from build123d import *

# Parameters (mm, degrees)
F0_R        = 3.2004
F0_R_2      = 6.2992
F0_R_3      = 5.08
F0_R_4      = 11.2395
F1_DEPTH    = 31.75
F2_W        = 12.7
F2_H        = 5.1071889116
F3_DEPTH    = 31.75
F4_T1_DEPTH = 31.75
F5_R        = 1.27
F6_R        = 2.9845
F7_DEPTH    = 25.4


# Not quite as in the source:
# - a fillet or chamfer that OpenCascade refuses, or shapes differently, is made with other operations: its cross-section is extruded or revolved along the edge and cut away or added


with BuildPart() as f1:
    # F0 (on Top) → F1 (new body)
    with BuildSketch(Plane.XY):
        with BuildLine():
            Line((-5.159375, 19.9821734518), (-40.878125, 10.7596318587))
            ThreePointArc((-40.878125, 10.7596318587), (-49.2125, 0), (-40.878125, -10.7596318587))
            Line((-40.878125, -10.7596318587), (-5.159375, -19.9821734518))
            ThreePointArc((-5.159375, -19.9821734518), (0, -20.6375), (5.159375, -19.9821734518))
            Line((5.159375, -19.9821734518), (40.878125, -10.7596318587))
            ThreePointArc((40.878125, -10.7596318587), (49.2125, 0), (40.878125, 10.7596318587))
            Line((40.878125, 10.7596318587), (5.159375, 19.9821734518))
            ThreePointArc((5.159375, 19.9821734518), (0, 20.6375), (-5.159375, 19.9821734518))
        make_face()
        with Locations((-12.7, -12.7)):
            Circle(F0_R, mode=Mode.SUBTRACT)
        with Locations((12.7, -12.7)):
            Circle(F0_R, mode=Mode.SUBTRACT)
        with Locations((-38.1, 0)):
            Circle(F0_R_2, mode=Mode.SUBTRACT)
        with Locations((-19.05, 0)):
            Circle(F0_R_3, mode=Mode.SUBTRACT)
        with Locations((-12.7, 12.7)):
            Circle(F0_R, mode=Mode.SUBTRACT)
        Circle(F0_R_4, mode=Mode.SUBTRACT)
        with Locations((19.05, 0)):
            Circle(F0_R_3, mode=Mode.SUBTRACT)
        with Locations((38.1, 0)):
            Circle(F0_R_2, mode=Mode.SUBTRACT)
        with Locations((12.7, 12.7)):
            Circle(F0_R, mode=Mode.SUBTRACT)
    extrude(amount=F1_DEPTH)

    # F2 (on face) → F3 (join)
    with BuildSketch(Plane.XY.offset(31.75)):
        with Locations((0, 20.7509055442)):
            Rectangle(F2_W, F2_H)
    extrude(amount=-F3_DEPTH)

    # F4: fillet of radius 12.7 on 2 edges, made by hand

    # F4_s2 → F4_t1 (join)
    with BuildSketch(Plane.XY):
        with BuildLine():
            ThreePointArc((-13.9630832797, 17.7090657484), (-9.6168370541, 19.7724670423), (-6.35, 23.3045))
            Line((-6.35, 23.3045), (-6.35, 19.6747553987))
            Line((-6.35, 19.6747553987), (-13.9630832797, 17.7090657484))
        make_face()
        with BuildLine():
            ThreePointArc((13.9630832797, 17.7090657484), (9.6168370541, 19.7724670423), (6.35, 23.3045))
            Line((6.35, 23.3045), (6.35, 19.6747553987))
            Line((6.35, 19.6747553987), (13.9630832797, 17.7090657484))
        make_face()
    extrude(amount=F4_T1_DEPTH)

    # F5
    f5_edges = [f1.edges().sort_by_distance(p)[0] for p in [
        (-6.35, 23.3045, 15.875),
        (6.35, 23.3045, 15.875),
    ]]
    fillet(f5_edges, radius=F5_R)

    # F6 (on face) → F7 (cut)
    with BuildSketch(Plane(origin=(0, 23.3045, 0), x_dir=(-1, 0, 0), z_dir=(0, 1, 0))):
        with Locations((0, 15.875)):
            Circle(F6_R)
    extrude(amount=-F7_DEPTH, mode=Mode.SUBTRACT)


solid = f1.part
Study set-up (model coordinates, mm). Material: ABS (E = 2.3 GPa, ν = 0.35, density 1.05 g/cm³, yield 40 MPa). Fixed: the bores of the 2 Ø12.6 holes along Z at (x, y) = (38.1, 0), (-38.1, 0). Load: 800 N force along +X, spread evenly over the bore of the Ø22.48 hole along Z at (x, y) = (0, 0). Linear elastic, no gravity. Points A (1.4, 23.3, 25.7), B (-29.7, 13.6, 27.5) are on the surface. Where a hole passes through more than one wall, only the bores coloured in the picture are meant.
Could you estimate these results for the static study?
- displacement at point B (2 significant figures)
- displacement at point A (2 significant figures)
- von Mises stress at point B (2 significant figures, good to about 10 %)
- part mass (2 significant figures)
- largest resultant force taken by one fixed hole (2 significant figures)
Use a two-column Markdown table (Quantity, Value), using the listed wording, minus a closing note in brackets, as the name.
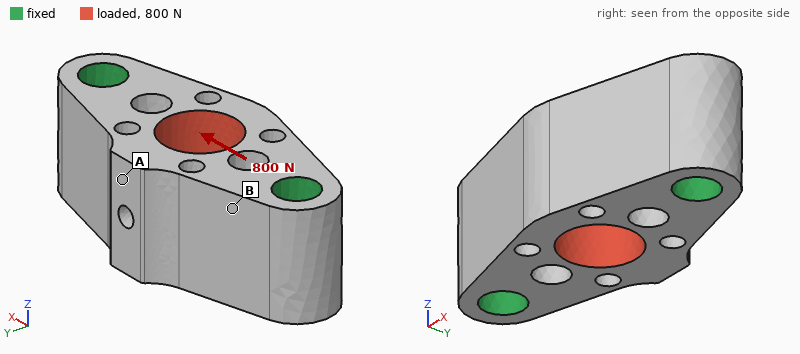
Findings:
| Quantity | Value |
|---|---|
| displacement at point B | 3.9 µm |
| displacement at point A | 5.6 µm |
| von Mises stress at point B | 0.43 MPa |
| part mass | 66 g |
| largest resultant force taken by one fixed hole | 400 N |
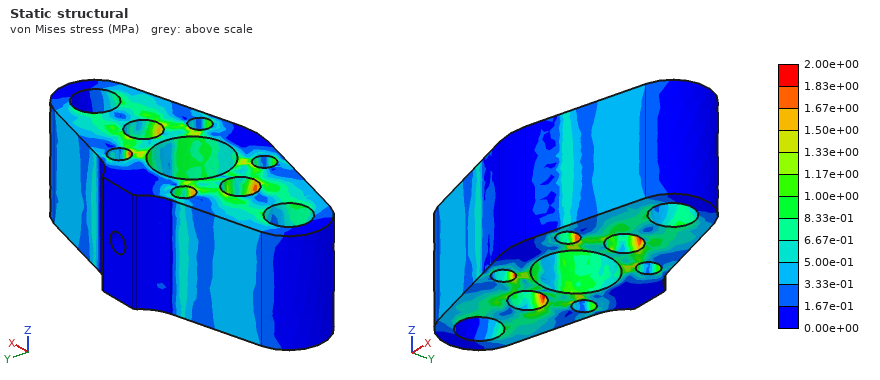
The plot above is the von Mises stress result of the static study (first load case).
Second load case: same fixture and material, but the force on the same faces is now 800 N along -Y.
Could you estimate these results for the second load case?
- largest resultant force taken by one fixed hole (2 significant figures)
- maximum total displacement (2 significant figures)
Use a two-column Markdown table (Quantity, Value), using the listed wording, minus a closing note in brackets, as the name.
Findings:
| Quantity | Value |
|---|---|
| largest resultant force taken by one fixed hole | 400 N |
| maximum total displacement | 41 µm |
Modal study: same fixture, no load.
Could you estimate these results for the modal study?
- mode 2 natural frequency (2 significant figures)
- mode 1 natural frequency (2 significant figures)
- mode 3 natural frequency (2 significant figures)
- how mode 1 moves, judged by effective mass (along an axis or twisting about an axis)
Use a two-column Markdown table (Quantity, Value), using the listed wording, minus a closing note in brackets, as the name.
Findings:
| Quantity | Value |
|---|---|
| mode 2 natural frequency | 4600 Hz |
| mode 1 natural frequency | 4300 Hz |
| mode 3 natural frequency | 4800 Hz |
| how mode 1 moves, judged by effective mass | along Z |
